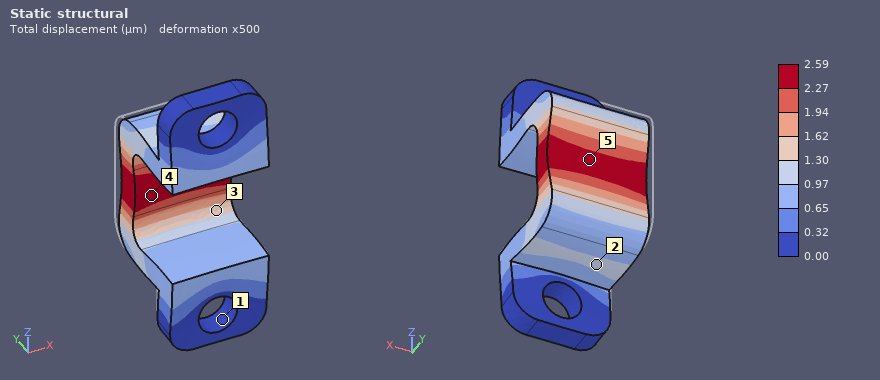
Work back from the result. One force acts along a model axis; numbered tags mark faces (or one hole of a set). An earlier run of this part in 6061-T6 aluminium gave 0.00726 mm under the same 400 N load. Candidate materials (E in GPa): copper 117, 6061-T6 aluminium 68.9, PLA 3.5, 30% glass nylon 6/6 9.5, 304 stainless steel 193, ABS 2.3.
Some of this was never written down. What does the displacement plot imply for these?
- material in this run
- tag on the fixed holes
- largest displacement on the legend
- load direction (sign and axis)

304 stainless steel
1
2.59 µm
-Y
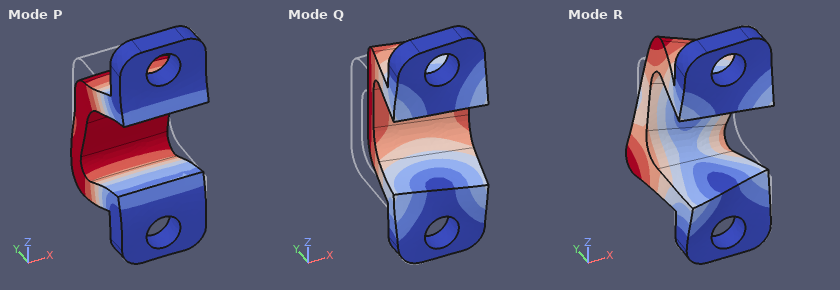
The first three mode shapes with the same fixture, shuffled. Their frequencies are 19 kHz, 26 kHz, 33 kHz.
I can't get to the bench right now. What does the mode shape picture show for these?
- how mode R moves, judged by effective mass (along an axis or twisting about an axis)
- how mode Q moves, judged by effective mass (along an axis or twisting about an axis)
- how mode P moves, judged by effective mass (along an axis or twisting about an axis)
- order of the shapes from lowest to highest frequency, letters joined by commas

twisting about Y
along X
along Z
Q, P, R
